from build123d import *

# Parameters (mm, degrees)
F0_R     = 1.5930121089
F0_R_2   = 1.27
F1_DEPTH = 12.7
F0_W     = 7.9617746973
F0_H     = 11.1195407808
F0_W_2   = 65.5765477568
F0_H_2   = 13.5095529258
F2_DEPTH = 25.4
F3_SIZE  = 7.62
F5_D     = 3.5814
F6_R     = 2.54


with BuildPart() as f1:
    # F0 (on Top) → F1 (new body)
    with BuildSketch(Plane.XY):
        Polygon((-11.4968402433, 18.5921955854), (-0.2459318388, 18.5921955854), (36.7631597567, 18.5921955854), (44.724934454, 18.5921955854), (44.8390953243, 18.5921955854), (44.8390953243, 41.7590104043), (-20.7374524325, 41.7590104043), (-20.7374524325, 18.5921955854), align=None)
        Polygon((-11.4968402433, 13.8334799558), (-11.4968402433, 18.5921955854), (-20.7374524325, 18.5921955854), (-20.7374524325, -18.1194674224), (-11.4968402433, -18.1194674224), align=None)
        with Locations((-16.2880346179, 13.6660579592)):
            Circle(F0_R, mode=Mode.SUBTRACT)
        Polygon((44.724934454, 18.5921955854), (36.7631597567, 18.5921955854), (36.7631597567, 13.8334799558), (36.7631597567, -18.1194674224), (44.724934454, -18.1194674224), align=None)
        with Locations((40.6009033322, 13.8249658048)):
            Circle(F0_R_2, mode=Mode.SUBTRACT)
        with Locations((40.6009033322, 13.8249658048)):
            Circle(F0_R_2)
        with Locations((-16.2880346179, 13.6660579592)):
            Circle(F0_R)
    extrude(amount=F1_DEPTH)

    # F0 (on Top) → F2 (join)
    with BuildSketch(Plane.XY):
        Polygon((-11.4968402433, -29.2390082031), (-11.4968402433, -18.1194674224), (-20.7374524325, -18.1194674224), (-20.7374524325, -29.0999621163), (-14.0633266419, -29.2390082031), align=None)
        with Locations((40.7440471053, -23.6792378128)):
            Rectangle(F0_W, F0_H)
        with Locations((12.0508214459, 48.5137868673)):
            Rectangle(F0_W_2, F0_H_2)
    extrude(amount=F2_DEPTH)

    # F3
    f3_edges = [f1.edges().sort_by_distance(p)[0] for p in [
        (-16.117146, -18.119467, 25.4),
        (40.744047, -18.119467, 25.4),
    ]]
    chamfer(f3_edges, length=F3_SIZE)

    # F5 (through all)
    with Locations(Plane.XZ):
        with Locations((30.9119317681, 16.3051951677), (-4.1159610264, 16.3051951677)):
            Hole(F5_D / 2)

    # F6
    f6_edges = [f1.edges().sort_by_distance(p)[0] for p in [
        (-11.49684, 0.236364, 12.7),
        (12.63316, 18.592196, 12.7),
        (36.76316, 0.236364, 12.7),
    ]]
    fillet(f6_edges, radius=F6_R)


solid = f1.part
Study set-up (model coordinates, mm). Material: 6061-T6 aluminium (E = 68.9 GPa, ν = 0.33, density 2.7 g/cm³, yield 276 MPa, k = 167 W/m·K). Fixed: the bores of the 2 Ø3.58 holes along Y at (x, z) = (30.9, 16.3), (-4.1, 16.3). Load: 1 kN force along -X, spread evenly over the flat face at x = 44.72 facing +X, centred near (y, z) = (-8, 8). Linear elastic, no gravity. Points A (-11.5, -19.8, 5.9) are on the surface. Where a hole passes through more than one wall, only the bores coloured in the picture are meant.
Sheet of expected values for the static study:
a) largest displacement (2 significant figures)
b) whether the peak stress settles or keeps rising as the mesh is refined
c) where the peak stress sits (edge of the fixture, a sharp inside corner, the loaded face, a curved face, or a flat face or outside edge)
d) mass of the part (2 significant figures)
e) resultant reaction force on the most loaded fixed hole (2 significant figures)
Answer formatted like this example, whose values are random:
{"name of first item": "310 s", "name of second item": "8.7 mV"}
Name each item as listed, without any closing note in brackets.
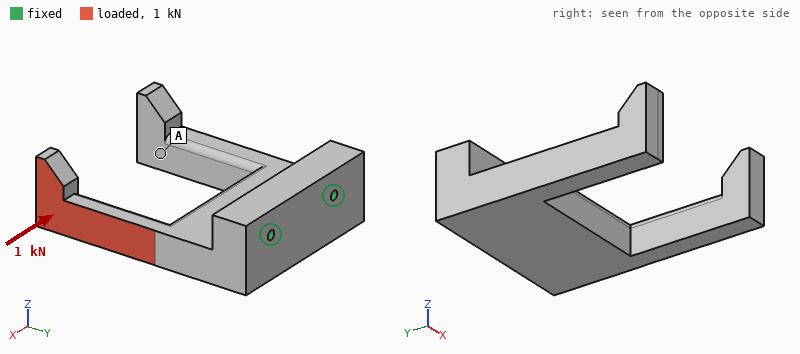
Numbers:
{"largest displacement": "0.74 mm", "whether the peak stress settles or keeps rising as the mesh is refined": "keeps rising", "where the peak stress sits": "a sharp inside corner", "mass of the part": "150 g", "resultant reaction force on the most loaded fixed hole": "1.5 kN"}
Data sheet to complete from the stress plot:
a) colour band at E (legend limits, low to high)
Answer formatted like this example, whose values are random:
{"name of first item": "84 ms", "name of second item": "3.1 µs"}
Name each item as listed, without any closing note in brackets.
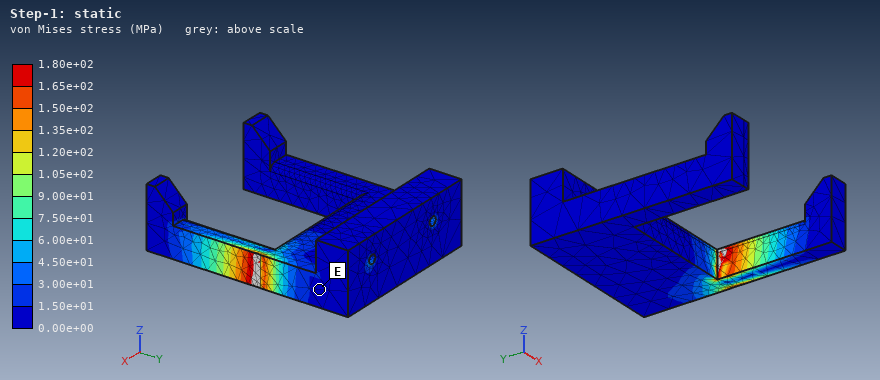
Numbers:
{"colour band at E": "0.00e+00 to 1.50e+01 MPa"}
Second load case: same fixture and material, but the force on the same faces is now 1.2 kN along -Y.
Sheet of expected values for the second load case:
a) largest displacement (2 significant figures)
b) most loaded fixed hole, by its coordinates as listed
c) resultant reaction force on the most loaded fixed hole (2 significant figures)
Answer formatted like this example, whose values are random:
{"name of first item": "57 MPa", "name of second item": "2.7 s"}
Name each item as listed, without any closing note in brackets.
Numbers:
{"largest displacement": "0.17 mm", "most loaded fixed hole, by its coordinates as listed": "(30.9, 16.3)", "resultant reaction force on the most loaded fixed hole": "1.5 kN"}
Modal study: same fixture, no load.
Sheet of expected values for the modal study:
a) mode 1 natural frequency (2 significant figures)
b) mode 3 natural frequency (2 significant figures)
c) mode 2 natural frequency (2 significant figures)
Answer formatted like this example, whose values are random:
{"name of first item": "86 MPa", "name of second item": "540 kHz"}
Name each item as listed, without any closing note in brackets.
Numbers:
{"mode 1 natural frequency": "1800 Hz", "mode 3 natural frequency": "2000 Hz", "mode 2 natural frequency": "1800 Hz"}
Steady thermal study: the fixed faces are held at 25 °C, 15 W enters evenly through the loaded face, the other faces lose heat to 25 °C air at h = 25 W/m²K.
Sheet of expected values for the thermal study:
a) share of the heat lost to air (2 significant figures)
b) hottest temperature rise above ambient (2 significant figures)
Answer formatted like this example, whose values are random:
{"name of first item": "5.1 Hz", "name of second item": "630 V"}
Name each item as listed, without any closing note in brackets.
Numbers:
{"share of the heat lost to air": "11 %", "hottest temperature rise above ambient": "34 K"}
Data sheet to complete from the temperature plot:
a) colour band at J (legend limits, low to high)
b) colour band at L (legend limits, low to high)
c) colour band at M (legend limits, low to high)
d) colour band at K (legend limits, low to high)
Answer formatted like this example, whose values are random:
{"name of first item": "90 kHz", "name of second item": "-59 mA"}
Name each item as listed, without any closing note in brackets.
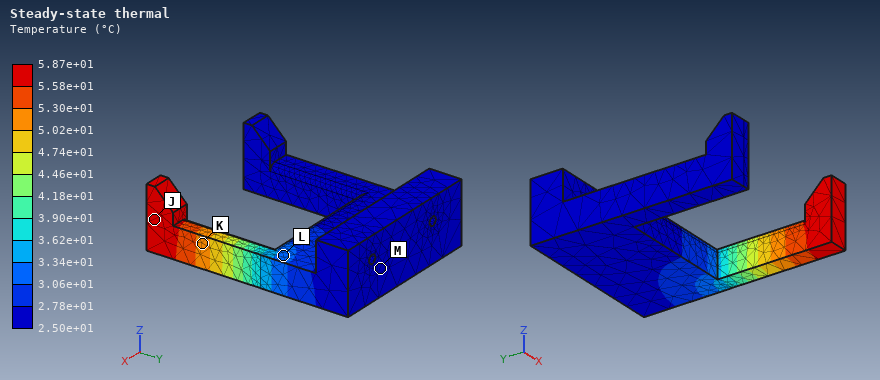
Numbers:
{"colour band at J": "5.58e+01 to 5.87e+01 °C", "colour band at L": "3.06e+01 to 3.34e+01 °C", "colour band at M": "2.50e+01 to 2.78e+01 °C", "colour band at K": "5.02e+01 to 5.30e+01 °C"}
